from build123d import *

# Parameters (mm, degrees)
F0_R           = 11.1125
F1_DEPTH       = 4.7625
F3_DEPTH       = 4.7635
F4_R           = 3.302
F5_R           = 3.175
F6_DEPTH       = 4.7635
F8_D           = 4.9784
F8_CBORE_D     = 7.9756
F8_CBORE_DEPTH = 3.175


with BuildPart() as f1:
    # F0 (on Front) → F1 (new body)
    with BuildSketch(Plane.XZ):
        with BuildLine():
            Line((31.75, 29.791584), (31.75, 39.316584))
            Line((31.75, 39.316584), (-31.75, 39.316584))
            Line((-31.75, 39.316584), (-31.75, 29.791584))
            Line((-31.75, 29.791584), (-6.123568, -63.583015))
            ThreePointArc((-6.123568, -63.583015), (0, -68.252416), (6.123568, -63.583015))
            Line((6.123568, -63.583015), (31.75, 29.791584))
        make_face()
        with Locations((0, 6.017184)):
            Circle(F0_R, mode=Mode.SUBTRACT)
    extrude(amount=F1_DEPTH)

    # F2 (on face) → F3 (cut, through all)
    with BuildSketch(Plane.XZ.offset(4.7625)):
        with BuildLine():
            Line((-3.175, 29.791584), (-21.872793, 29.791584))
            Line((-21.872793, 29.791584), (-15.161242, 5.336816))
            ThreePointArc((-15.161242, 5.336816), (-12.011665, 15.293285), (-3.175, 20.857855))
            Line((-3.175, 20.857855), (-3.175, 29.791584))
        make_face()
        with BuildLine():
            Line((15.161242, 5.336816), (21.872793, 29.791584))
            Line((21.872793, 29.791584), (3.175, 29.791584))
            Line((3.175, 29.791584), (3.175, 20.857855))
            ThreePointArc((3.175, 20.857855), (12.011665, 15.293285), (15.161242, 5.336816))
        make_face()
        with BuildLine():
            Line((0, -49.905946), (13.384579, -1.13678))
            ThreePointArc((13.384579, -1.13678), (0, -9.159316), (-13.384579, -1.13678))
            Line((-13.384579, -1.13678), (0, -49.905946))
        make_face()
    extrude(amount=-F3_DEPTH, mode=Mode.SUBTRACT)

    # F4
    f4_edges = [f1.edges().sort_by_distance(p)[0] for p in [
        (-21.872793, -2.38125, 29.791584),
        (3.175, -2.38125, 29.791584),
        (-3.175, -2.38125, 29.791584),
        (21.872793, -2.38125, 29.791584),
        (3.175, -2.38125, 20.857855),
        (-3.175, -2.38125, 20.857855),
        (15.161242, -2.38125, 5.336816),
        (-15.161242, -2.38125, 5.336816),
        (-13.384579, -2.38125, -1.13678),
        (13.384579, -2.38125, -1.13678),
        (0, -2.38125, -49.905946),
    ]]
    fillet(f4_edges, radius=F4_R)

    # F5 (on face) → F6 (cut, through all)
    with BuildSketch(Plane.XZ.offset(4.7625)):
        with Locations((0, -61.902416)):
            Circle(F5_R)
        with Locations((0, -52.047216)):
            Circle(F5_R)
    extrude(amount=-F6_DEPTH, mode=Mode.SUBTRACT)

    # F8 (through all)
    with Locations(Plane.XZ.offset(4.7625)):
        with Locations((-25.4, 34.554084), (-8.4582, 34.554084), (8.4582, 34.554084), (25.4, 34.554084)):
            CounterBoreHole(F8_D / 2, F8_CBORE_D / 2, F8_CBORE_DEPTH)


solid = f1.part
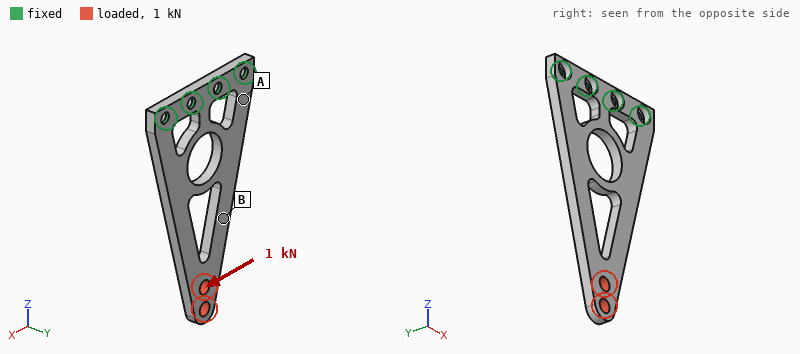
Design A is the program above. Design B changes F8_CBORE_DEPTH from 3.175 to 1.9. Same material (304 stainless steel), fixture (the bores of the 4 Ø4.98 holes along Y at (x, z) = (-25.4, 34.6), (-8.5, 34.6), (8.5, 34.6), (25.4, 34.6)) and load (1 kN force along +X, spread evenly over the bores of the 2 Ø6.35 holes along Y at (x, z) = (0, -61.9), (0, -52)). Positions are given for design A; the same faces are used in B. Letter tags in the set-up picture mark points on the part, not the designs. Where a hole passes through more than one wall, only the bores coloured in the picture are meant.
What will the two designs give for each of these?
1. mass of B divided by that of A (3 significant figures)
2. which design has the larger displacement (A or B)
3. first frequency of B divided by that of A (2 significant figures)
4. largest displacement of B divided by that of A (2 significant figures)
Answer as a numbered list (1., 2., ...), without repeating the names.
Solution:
1. 1.01
2. A
3. 1.1
4. 0.89
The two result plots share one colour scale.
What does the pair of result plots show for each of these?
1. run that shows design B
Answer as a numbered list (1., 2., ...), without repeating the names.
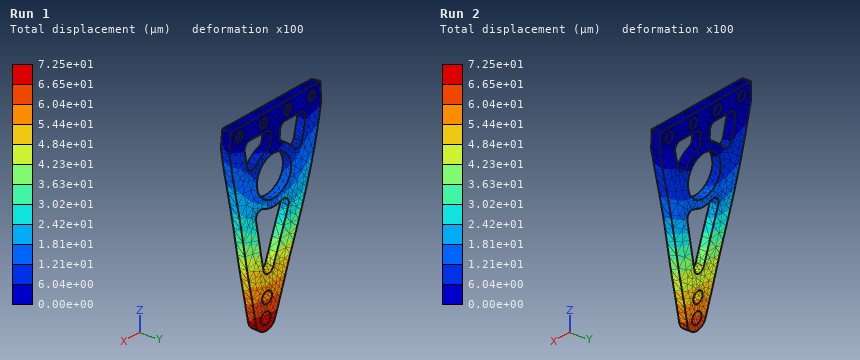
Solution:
1. Run 2
